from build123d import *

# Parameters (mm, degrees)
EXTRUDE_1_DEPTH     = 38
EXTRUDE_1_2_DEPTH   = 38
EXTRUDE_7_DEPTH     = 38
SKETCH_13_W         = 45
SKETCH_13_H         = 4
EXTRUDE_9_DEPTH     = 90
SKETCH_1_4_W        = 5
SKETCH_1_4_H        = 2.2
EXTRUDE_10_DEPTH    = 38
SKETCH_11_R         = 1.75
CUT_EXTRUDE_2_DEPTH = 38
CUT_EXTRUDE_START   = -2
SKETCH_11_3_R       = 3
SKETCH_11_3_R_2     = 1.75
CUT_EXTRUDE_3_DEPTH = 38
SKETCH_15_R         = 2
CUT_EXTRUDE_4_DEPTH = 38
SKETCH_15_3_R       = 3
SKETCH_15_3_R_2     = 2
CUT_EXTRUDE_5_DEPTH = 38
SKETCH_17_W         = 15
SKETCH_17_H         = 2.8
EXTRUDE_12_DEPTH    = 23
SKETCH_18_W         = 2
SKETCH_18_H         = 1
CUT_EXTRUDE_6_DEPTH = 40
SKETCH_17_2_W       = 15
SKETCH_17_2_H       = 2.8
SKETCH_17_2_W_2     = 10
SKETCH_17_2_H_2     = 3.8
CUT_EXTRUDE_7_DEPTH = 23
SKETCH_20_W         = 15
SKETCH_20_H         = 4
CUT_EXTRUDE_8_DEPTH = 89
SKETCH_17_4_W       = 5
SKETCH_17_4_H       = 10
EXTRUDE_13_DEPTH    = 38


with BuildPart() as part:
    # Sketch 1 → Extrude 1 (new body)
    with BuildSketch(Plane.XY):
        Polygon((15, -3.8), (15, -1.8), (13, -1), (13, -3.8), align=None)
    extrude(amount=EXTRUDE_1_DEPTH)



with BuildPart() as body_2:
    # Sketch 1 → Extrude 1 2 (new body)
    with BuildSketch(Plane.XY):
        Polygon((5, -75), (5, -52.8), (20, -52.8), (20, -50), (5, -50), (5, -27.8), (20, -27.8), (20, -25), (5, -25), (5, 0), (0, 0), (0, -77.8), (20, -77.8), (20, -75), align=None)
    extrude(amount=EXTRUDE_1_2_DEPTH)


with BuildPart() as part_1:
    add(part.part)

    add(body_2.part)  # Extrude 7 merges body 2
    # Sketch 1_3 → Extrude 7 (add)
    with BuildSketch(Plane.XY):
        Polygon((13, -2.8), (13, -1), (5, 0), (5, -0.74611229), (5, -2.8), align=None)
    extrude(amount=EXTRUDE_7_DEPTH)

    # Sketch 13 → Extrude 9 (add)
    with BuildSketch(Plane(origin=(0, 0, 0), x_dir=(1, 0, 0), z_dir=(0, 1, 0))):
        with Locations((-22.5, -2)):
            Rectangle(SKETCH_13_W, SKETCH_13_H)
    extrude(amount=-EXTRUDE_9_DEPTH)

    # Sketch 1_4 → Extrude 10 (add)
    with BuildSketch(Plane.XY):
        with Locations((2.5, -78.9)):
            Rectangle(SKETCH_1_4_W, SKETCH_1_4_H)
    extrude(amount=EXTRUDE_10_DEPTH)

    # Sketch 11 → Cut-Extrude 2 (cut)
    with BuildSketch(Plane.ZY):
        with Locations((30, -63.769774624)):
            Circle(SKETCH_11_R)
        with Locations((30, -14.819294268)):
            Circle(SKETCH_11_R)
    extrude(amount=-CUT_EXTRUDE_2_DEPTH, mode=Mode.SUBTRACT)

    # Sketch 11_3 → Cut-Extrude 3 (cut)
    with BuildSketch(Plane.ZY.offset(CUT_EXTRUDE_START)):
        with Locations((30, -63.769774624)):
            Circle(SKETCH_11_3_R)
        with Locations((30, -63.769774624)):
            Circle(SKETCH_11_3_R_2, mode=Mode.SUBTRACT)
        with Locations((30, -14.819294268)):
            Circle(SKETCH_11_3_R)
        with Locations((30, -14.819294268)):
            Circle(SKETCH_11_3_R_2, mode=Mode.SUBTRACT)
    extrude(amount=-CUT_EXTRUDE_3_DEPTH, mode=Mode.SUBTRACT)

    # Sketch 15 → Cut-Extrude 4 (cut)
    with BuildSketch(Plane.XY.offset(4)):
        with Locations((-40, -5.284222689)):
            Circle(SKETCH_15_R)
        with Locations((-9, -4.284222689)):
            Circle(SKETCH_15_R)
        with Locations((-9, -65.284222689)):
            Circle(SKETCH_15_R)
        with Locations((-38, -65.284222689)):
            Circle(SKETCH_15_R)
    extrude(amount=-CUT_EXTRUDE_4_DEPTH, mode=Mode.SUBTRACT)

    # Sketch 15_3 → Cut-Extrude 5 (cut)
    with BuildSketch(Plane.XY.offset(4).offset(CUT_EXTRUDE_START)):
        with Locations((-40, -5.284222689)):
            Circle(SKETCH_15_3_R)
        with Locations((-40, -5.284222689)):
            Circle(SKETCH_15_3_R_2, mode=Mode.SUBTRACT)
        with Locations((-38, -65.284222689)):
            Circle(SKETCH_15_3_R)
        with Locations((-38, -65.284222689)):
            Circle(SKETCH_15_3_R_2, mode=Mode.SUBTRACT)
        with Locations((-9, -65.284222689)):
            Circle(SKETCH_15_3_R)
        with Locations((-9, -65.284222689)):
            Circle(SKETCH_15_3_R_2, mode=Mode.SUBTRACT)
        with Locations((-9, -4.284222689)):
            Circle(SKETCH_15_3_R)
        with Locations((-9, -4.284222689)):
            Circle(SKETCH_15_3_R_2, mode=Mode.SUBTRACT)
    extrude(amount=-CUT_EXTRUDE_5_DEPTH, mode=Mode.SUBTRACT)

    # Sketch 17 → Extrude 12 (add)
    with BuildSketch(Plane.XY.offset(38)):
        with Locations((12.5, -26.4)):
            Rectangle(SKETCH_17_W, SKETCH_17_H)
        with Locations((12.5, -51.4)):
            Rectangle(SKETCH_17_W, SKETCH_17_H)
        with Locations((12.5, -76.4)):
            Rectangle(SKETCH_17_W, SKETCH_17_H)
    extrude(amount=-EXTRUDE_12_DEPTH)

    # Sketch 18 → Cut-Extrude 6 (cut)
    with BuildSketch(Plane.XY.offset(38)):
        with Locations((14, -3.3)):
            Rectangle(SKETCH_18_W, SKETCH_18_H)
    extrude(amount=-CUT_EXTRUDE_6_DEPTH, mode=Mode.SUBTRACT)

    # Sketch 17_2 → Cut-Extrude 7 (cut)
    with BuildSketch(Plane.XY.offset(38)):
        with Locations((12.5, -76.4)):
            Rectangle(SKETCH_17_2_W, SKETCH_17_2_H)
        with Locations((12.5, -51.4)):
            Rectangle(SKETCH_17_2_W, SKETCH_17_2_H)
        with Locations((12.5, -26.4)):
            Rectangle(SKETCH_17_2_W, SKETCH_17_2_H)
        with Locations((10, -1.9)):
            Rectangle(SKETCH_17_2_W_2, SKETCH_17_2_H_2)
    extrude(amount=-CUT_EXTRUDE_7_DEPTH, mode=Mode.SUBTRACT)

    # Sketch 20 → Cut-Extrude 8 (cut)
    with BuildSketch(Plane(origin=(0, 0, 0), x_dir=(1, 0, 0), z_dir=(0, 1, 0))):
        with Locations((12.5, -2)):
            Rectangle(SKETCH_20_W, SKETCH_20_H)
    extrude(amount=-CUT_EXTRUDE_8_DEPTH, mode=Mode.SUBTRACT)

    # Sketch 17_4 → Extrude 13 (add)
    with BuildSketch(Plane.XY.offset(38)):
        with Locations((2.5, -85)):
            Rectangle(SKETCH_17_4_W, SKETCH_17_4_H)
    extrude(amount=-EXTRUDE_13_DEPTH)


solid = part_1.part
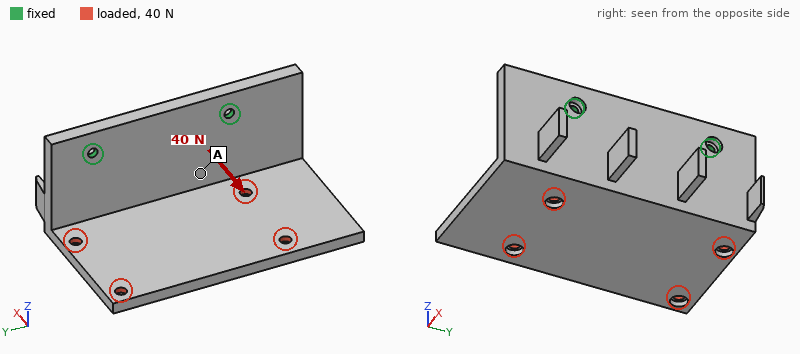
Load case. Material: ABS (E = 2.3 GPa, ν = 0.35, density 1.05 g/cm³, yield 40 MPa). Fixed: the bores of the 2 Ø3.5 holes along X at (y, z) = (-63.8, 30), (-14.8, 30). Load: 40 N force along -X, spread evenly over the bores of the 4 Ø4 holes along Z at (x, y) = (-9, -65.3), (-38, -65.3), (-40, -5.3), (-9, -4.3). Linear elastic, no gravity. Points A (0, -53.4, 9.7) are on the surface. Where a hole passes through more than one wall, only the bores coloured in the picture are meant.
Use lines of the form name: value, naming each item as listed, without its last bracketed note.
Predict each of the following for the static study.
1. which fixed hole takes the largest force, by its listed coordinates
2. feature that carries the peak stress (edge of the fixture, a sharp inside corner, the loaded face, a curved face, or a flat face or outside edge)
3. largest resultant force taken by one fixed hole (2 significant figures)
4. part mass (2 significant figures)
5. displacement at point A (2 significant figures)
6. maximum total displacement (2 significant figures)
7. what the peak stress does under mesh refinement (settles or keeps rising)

which fixed hole takes the largest force, by its listed coordinates: (-14.8, 30)
feature that carries the peak stress: edge of the fixture
largest resultant force taken by one fixed hole: 23 N
part mass: 36 g
displacement at point A: 0.41 mm
maximum total displacement: 1.3 mm
what the peak stress does under mesh refinement: keeps rising
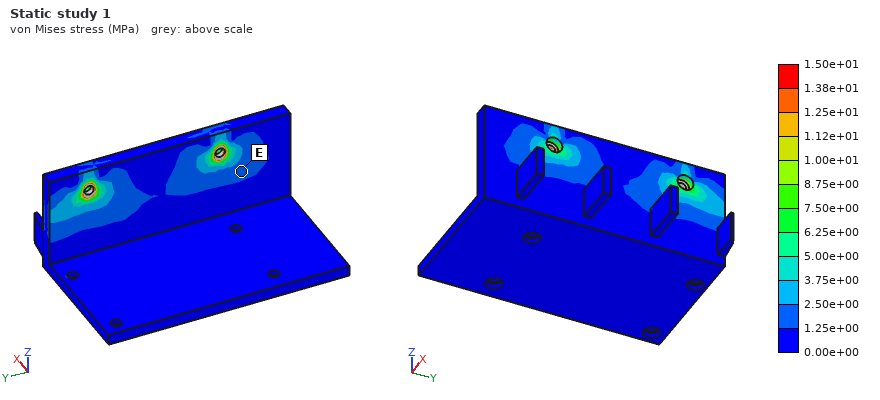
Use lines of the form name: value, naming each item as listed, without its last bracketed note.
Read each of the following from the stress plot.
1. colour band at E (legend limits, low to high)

colour band at E: 1.25e+00 to 2.50e+00 MPa
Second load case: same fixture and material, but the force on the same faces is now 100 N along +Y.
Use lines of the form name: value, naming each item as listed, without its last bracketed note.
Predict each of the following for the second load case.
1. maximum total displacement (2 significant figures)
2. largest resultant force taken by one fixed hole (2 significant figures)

maximum total displacement: 1.2 mm
largest resultant force taken by one fixed hole: 90 N
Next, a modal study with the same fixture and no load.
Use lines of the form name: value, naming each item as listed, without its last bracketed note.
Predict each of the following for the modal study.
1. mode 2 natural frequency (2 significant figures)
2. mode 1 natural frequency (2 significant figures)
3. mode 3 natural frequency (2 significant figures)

mode 2 natural frequency: 370 Hz
mode 1 natural frequency: 190 Hz
mode 3 natural frequency: 540 Hz
